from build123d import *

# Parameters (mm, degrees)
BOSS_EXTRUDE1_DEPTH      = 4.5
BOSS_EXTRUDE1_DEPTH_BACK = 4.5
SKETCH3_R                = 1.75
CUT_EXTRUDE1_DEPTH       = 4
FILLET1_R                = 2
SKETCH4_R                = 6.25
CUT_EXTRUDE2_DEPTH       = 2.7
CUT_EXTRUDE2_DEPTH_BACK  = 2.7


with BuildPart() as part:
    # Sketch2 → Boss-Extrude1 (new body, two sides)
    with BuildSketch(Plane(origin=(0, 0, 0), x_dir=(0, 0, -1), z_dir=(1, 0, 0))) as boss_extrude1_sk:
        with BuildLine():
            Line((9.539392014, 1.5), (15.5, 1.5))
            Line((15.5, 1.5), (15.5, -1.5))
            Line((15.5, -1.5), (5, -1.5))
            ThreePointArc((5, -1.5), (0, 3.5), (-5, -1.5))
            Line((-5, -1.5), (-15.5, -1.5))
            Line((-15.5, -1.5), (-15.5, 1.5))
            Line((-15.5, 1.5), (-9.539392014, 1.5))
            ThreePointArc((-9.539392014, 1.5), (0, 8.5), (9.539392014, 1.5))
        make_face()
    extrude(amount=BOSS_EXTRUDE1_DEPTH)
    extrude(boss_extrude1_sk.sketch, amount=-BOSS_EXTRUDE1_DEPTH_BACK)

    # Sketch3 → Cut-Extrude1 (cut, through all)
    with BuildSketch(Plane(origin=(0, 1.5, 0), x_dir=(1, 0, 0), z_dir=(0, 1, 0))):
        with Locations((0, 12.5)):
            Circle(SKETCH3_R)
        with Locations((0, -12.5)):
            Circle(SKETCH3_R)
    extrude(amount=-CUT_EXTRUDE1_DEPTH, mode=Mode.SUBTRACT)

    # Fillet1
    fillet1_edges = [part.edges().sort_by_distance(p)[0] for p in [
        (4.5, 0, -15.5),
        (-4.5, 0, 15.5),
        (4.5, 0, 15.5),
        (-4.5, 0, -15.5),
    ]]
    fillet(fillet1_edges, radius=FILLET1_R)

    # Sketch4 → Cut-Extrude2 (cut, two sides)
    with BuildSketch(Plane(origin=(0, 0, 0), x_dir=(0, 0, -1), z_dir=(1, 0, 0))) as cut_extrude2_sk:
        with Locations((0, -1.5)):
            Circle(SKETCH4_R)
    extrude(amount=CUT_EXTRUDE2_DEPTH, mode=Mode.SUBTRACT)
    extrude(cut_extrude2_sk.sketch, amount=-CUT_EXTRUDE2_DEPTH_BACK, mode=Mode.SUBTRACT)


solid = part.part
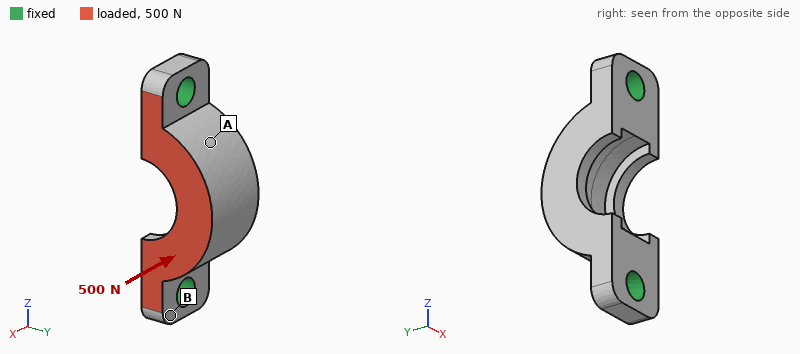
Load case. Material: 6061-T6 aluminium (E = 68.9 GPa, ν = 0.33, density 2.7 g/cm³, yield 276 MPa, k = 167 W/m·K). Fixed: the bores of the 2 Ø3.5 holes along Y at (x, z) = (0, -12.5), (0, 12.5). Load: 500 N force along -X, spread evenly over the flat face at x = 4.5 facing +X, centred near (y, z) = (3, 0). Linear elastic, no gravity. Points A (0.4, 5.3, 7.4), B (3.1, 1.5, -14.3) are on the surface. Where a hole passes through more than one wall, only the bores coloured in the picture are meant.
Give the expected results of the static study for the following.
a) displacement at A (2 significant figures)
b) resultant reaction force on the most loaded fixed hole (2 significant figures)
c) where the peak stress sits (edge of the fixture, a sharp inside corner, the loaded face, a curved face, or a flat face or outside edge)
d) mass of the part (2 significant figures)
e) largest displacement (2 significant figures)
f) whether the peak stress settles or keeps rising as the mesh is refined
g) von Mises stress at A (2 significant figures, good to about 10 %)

8.7 µm
250 N
edge of the fixture
3.2 g
16 µm
keeps rising
17 MPa
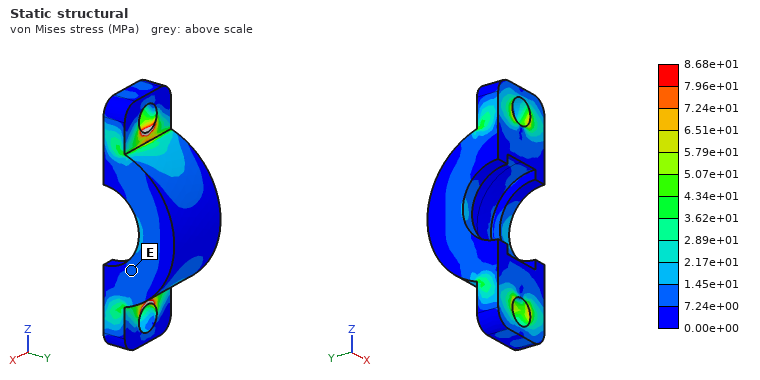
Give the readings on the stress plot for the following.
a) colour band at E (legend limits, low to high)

7.24e+00 to 1.45e+01 MPa
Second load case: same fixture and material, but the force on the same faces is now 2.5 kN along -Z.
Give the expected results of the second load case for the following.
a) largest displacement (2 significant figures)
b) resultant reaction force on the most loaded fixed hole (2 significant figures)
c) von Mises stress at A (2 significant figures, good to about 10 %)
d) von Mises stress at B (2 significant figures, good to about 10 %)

19 µm
1.3 kN
27 MPa
39 MPa
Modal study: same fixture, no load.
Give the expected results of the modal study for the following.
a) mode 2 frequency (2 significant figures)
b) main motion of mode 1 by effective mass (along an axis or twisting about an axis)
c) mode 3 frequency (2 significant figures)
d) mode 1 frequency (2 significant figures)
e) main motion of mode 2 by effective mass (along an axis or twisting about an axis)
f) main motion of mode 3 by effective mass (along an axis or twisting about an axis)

40 kHz
along X
52 kHz
19 kHz
along Y
along Z
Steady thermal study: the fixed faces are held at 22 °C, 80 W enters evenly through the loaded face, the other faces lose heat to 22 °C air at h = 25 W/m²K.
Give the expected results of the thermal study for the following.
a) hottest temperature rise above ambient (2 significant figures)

62 K
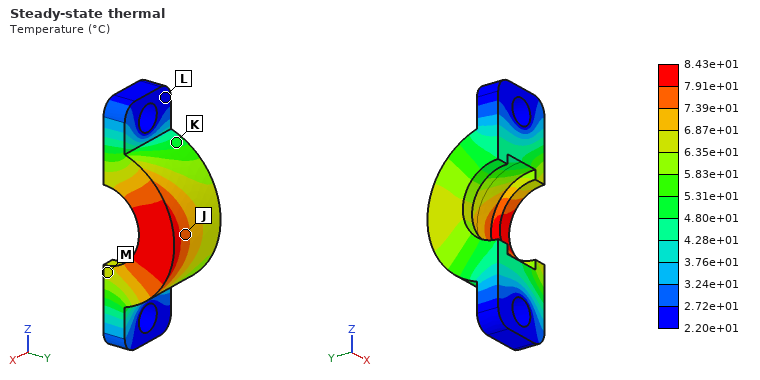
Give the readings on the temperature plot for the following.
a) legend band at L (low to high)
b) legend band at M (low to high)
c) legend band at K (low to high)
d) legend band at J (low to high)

2.20e+01 to 2.72e+01 °C
6.35e+01 to 6.87e+01 °C
4.80e+01 to 5.31e+01 °C
7.39e+01 to 7.91e+01 °C
